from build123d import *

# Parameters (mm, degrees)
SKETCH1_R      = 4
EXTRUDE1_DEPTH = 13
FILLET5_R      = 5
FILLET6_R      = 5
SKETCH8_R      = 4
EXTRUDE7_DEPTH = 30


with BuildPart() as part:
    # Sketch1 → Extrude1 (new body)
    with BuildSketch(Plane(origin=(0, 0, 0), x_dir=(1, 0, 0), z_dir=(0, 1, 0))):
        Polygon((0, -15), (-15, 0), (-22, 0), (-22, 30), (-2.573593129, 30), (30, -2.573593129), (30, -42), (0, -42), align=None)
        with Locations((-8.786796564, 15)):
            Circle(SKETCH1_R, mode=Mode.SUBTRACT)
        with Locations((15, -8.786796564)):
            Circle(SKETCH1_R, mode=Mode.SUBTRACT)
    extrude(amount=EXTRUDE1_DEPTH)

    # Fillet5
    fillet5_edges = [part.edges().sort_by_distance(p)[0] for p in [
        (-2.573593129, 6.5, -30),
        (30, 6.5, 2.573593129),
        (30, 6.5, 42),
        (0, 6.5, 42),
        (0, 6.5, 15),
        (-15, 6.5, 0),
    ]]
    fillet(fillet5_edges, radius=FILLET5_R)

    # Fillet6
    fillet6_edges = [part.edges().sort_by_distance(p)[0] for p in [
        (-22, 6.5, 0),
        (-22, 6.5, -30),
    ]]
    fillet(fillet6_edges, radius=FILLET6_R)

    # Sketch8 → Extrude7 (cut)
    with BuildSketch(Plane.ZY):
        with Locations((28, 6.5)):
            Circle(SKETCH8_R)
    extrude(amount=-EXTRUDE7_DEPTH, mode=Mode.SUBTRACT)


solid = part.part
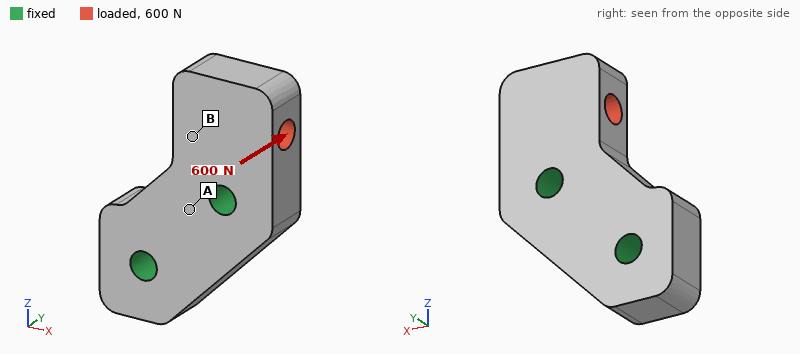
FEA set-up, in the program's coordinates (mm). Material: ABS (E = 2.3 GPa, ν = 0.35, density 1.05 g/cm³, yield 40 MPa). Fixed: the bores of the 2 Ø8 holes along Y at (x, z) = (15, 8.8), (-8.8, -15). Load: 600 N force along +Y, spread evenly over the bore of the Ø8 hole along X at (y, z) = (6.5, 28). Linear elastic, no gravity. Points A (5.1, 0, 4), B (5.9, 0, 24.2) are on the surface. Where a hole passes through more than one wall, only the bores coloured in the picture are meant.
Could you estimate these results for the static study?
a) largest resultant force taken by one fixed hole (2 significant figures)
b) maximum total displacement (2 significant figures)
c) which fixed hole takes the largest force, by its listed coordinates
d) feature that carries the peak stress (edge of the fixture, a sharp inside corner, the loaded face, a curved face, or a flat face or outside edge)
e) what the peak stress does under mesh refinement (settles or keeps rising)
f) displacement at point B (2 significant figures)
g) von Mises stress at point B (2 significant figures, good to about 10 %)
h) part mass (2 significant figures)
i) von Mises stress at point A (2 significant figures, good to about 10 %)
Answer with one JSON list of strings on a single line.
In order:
["650 N", "0.32 mm", "(15, 8.8)", "edge of the fixture", "keeps rising", "0.12 mm", "7.5 MPa", "30 g", "2.6 MPa"]
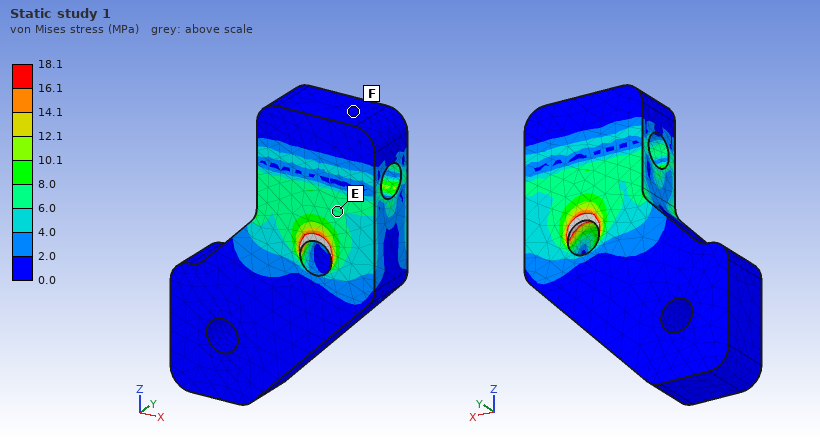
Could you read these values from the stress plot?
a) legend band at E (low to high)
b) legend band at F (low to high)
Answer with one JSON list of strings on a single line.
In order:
["6.0 to 8.0 MPa", "0.0 to 2.0 MPa"]
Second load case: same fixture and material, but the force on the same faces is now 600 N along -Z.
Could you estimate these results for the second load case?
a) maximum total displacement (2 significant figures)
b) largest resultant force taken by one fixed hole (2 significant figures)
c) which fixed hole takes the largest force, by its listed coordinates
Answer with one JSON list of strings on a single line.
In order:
["27 µm", "540 N", "(15, 8.8)"]
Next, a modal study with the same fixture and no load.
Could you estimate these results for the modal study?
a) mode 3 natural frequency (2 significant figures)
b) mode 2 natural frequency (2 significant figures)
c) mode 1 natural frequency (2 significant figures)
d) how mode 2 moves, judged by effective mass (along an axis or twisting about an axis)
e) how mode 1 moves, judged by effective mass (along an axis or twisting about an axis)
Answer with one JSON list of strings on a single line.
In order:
["4700 Hz", "3700 Hz", "2500 Hz", "along X", "along Y"]
